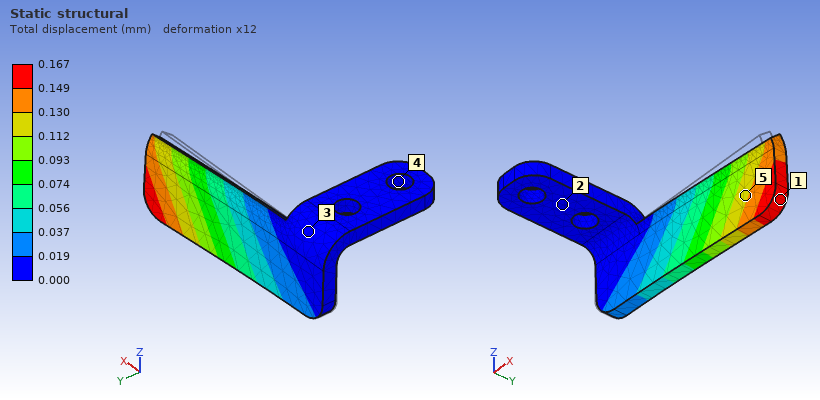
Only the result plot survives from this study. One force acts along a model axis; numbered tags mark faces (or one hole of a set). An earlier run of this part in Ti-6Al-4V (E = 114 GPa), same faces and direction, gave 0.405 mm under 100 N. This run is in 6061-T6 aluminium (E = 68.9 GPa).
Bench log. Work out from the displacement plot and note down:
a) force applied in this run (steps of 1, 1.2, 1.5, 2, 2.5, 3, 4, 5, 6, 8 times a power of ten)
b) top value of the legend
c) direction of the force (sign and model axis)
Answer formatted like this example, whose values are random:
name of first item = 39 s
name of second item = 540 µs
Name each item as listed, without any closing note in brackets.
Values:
force applied in this run = 25 N
top value of the legend = 0.167 mm
direction of the force = +Y
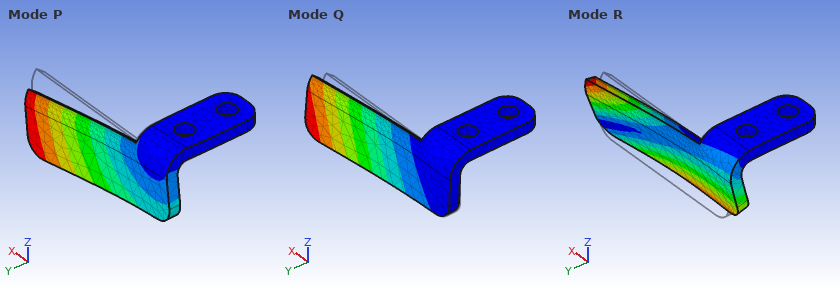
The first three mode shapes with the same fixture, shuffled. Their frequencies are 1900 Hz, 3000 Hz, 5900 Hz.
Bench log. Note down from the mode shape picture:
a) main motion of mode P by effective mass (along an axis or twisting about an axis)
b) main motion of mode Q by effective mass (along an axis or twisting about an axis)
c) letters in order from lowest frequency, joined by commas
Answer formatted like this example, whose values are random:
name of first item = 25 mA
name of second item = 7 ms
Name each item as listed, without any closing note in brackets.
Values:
main motion of mode P by effective mass = along Z
main motion of mode Q by effective mass = along Y
letters in order from lowest frequency, joined by commas = Q, P, R
